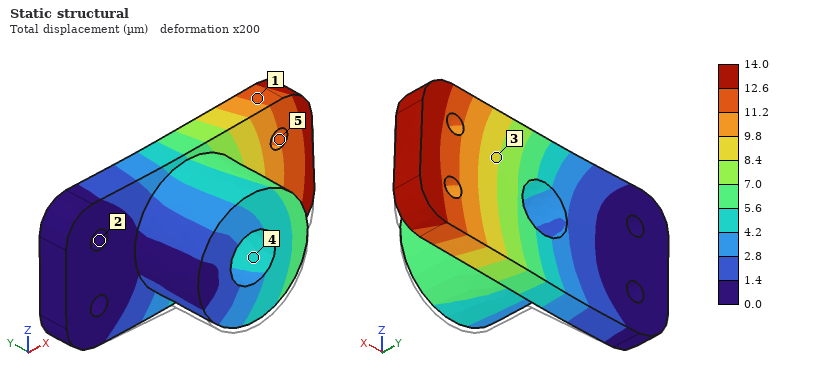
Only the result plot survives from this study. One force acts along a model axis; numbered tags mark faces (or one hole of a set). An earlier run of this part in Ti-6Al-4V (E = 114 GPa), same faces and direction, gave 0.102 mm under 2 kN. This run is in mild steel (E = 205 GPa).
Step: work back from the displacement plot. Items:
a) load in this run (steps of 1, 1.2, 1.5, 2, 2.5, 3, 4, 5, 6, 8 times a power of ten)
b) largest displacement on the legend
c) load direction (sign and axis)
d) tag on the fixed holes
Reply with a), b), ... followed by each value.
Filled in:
a) 500 N
b) 14.0 µm
c) +Z
d) 2
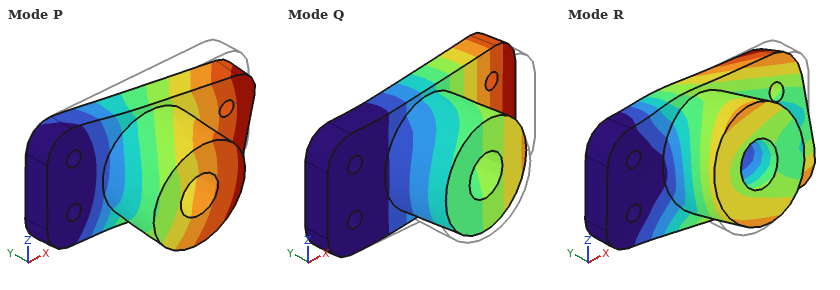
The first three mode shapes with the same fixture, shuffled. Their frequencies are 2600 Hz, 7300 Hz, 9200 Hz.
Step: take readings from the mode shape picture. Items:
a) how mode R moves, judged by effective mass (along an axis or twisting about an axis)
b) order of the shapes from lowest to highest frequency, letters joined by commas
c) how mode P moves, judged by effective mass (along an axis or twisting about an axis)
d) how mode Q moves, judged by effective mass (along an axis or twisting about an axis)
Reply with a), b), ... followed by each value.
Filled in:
a) twisting about X
b) Q, P, R
c) along Z
d) along Y
